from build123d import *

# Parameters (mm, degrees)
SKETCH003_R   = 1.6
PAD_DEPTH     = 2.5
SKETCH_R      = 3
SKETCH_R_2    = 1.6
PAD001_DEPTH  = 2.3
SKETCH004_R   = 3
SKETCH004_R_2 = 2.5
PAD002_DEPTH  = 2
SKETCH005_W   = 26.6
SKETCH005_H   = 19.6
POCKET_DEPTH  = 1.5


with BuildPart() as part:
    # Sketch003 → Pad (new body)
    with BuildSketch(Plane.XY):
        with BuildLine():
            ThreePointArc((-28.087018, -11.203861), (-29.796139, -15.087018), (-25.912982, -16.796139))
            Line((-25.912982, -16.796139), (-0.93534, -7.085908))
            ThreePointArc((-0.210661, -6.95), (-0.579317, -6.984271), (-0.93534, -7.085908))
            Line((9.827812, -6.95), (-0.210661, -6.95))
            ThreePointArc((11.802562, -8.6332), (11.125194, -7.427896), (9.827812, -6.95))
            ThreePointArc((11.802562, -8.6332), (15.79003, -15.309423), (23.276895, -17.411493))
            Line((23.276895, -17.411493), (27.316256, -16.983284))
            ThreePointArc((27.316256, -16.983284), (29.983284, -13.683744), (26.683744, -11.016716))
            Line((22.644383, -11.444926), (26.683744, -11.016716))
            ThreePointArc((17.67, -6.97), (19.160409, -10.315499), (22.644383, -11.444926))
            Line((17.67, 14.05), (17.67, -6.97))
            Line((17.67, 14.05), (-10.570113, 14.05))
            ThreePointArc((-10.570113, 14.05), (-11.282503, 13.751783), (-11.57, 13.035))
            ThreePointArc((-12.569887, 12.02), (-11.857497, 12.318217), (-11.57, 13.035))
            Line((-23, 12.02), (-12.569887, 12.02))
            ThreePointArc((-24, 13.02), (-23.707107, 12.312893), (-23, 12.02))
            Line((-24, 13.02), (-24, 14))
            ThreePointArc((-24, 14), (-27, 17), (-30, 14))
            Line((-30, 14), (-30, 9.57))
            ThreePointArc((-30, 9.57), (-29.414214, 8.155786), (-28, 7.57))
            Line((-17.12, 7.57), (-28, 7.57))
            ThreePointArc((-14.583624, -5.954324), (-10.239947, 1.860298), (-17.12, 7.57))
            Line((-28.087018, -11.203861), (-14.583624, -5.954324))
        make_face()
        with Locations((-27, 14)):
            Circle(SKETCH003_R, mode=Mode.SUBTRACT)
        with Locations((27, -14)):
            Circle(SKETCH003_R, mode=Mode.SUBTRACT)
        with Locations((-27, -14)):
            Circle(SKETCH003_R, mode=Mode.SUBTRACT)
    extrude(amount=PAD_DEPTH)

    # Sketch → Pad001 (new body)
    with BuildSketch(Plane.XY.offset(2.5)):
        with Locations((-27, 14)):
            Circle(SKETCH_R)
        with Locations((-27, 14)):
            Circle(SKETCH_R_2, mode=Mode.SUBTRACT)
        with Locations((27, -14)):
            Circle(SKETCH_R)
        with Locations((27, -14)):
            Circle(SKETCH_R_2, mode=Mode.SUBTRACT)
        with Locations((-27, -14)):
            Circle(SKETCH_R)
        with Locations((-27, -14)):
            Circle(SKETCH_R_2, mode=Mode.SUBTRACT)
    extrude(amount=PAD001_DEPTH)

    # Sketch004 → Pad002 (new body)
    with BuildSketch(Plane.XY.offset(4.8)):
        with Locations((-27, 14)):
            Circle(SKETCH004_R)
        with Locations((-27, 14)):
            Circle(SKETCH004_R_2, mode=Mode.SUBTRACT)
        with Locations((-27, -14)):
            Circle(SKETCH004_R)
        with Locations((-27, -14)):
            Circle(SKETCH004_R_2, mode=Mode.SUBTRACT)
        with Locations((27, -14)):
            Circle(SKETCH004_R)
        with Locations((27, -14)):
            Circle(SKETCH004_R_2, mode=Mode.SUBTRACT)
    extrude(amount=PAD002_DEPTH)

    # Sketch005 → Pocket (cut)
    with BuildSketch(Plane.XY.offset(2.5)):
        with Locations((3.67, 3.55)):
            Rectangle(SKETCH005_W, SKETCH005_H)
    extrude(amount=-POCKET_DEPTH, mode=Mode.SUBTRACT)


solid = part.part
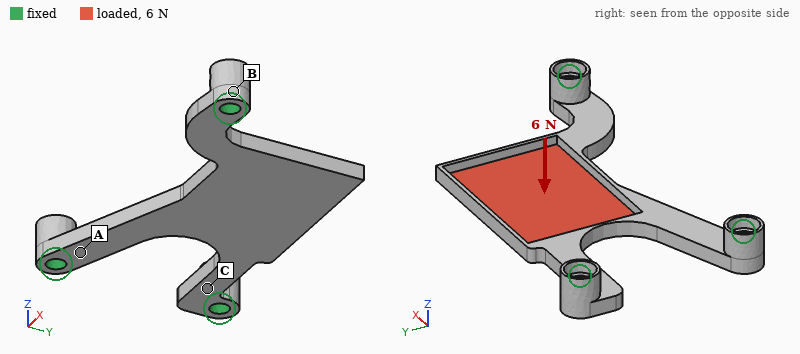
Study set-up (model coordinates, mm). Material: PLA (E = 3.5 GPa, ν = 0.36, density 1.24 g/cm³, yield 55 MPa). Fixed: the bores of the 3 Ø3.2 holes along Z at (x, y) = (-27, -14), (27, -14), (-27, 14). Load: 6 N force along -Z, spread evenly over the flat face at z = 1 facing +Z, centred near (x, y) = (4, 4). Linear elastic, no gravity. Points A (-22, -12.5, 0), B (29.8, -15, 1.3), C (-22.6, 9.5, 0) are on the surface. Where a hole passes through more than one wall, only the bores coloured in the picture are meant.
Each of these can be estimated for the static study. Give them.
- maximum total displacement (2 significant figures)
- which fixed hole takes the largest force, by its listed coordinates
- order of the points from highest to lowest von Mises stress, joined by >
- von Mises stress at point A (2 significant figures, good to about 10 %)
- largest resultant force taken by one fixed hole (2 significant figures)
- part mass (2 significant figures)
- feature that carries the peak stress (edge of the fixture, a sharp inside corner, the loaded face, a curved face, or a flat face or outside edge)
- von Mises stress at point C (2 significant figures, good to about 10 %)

0.64 mm
(-27, 14)
C > A > B
3.2 MPa
8.8 N
2.2 g
a curved face
5.5 MPa
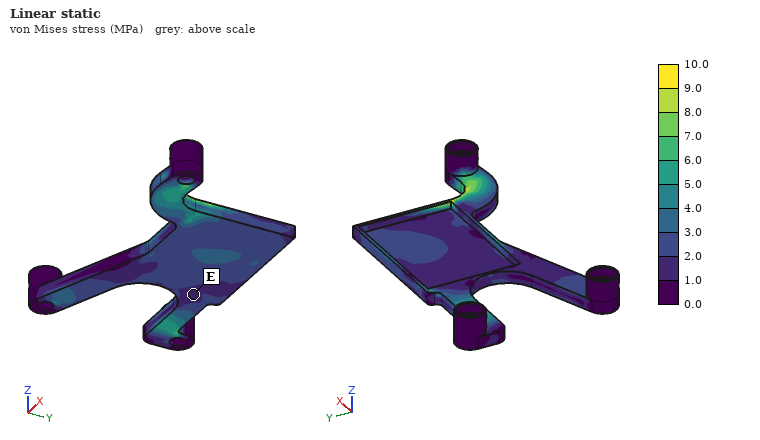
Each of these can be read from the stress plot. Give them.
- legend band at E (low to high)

1.0 to 2.0 MPa
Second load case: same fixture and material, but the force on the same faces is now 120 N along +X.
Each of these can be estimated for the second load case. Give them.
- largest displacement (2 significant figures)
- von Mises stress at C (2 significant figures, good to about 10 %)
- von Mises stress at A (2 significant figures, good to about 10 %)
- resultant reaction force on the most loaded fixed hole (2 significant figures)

0.16 mm
6.4 MPa
4.4 MPa
51 N
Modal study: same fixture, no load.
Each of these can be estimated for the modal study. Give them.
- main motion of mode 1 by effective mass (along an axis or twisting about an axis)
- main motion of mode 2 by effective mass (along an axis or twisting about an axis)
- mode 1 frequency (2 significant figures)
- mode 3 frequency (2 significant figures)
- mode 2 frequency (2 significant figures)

along Z
along Z
700 Hz
2100 Hz
1700 Hz
